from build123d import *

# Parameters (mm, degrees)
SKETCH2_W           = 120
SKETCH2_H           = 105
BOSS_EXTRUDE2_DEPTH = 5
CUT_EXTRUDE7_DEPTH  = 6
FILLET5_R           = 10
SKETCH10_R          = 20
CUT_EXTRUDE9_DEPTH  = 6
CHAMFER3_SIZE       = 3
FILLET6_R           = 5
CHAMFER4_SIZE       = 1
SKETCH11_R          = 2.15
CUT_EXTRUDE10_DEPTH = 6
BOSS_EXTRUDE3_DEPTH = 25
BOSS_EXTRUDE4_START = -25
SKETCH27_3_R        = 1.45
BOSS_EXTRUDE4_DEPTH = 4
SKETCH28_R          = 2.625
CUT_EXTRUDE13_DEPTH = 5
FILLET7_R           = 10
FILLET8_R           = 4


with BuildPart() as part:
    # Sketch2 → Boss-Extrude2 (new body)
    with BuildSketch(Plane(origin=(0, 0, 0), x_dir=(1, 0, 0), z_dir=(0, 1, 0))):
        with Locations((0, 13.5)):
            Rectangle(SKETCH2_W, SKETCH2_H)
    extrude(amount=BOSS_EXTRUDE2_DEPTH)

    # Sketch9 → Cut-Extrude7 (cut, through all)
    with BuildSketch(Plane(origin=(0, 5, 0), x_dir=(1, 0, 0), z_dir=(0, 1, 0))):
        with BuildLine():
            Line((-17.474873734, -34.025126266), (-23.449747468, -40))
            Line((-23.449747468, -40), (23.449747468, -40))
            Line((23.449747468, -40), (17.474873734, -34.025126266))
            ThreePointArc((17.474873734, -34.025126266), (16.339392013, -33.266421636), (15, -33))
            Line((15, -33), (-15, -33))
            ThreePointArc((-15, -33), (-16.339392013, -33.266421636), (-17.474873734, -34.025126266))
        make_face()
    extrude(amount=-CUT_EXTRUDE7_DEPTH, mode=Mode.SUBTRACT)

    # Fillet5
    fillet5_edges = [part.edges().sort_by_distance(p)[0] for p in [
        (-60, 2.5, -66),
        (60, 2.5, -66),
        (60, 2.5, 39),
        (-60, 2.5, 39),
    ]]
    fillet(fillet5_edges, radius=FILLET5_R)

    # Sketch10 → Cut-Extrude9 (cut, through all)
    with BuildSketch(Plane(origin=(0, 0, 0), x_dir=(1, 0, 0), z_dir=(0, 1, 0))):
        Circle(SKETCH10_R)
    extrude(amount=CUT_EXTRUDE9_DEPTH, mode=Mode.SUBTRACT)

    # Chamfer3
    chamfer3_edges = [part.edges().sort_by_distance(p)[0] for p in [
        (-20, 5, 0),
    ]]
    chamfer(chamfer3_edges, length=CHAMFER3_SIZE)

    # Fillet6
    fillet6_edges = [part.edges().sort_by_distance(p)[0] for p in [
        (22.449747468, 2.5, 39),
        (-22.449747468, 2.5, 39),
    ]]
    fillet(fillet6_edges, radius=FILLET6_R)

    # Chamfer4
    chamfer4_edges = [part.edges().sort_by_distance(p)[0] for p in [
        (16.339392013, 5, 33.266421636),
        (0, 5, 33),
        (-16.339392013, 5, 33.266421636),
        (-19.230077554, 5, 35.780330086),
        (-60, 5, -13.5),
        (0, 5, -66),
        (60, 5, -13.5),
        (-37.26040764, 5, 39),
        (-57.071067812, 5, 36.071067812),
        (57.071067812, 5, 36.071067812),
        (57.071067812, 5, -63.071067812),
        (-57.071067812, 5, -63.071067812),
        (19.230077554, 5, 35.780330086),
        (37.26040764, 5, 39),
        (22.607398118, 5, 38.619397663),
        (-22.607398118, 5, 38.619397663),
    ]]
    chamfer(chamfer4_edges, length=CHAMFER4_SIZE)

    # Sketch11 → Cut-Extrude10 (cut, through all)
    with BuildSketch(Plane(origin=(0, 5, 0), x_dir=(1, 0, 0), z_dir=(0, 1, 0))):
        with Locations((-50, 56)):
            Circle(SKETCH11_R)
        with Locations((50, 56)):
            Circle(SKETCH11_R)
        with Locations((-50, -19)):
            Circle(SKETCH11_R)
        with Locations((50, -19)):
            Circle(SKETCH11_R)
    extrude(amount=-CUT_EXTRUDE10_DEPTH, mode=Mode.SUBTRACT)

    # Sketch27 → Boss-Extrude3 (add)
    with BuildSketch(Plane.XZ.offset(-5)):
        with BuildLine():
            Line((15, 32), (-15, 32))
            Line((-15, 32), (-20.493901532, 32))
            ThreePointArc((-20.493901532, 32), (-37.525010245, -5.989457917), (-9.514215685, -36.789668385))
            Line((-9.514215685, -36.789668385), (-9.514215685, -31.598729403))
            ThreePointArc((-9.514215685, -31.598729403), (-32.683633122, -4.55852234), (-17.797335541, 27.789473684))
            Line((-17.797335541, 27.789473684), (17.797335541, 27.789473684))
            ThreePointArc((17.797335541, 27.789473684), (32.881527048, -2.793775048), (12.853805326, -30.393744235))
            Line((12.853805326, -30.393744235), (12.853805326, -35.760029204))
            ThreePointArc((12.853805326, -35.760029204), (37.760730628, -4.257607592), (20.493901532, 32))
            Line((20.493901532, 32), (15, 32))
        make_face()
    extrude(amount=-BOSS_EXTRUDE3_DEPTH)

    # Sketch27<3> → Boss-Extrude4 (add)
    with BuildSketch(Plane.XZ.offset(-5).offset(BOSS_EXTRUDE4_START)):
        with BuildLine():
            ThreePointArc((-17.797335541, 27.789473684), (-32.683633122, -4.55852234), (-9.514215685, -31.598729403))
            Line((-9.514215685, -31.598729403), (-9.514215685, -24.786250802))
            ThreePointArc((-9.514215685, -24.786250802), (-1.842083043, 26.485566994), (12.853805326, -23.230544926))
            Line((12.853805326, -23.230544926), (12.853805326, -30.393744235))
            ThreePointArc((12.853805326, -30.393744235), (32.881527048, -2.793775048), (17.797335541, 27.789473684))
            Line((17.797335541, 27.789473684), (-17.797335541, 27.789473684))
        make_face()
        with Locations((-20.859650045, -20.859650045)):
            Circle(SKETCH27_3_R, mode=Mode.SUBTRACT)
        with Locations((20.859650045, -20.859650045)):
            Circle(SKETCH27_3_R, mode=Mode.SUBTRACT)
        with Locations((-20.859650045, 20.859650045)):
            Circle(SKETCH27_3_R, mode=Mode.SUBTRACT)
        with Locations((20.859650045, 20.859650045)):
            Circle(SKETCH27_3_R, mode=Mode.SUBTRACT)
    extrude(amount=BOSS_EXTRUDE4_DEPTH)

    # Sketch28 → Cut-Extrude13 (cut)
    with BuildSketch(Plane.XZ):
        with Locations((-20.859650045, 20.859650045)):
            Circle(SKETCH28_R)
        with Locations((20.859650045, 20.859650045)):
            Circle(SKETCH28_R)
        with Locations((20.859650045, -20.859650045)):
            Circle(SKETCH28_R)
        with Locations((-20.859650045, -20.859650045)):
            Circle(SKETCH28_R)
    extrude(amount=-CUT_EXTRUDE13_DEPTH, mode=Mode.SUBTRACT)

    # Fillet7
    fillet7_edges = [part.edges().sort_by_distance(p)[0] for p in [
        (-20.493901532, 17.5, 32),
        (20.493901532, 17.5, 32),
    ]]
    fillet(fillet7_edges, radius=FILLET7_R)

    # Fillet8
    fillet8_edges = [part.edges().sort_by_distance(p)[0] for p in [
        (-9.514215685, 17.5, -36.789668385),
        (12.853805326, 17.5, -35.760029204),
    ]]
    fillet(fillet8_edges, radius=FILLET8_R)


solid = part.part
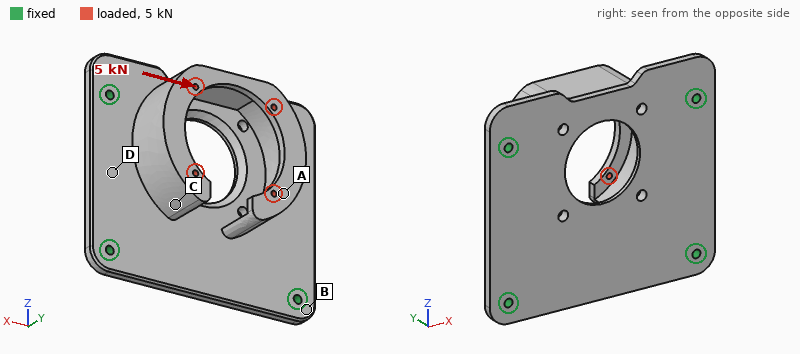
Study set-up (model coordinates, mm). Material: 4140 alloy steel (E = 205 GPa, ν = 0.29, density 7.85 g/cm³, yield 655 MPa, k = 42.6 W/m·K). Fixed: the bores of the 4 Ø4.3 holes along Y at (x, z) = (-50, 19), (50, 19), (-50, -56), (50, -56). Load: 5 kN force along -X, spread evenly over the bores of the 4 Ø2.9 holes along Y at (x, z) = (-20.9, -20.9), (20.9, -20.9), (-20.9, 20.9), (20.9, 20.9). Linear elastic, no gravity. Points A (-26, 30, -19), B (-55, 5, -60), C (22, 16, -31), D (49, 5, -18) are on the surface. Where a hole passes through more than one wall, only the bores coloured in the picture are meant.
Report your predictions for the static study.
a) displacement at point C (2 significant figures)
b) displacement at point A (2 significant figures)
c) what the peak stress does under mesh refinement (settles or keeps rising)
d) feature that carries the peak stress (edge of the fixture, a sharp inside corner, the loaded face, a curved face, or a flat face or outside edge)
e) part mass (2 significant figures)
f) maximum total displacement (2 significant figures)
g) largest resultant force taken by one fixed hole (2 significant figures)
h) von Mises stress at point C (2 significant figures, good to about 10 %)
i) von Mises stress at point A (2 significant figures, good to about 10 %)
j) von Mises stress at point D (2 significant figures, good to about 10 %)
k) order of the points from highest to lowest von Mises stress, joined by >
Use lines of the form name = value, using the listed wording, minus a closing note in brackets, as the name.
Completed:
displacement at point C = 17 µm
displacement at point A = 32 µm
what the peak stress does under mesh refinement = keeps rising
feature that carries the peak stress = edge of the fixture
part mass = 630 g
maximum total displacement = 46 µm
largest resultant force taken by one fixed hole = 2.2 kN
von Mises stress at point C = 32 MPa
von Mises stress at point A = 43 MPa
von Mises stress at point D = 16 MPa
order of the points from highest to lowest von Mises stress, joined by > = A > C > D > B
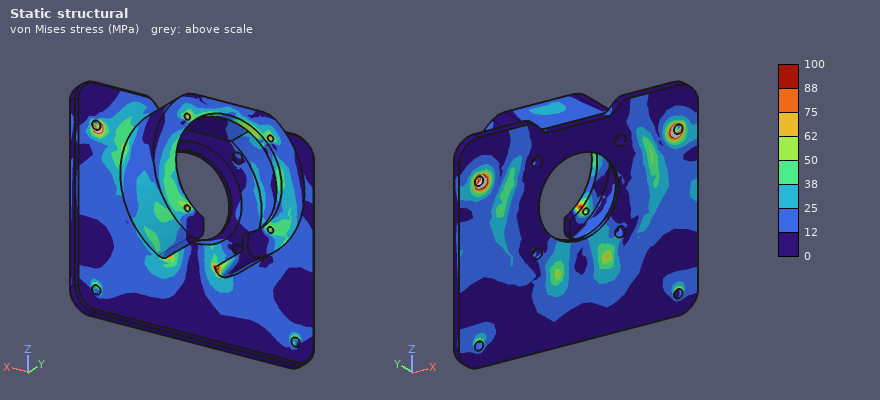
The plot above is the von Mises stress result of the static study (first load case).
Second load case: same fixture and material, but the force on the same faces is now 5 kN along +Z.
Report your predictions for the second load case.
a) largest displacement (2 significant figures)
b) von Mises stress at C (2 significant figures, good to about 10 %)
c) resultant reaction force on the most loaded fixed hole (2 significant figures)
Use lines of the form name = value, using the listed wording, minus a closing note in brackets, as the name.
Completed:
largest displacement = 87 µm
von Mises stress at C = 58 MPa
resultant reaction force on the most loaded fixed hole = 1.6 kN
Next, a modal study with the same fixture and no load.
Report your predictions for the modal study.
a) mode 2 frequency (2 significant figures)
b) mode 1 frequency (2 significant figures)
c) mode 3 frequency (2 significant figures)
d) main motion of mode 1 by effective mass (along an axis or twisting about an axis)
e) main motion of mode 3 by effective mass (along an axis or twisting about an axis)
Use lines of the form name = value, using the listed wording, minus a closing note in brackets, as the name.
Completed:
mode 2 frequency = 3000 Hz
mode 1 frequency = 2000 Hz
mode 3 frequency = 3900 Hz
main motion of mode 1 by effective mass = along Y
main motion of mode 3 by effective mass = twisting about Z
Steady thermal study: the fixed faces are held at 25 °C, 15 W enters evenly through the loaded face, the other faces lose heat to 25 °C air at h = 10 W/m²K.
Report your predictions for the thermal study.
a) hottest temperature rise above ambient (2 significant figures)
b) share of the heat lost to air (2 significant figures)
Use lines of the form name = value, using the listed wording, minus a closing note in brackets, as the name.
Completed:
hottest temperature rise above ambient = 31 K
share of the heat lost to air = 25 %
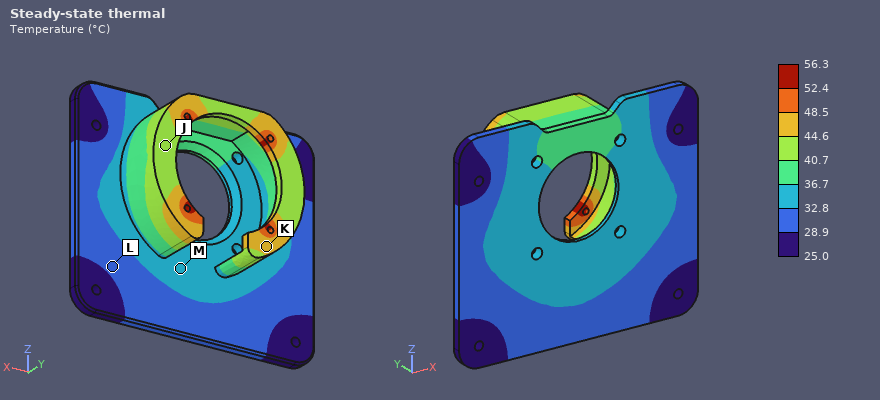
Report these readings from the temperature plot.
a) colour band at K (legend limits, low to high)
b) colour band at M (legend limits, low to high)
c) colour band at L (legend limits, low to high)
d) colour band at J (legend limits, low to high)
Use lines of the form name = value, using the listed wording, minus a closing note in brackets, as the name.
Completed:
colour band at K = 44.6 to 48.5 °C
colour band at M = 32.8 to 36.7 °C
colour band at L = 28.9 to 32.8 °C
colour band at J = 40.7 to 44.6 °C
